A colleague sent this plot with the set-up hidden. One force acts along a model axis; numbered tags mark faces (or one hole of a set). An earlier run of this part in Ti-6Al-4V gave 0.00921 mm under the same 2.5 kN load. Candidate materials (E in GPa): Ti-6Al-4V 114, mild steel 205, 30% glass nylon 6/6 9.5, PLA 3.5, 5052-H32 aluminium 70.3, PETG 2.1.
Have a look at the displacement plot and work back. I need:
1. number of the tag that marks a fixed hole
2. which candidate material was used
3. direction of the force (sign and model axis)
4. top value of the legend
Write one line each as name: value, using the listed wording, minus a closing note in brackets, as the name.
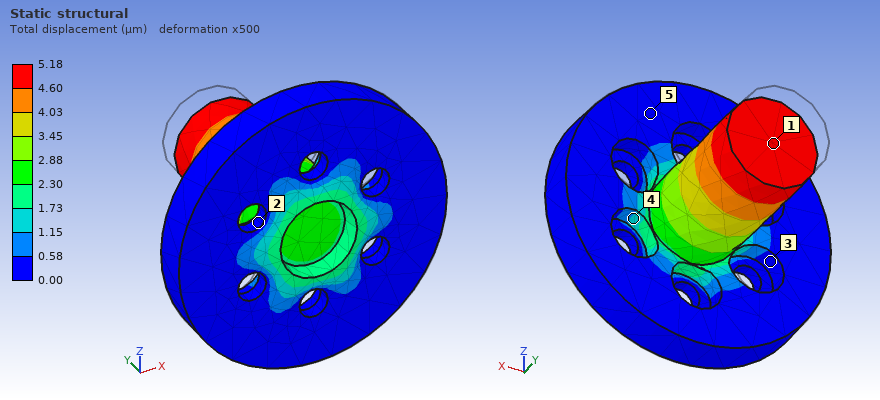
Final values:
number of the tag that marks a fixed hole: 2
which candidate material was used: mild steel
direction of the force: -Y
top value of the legend: 5.18 µm
